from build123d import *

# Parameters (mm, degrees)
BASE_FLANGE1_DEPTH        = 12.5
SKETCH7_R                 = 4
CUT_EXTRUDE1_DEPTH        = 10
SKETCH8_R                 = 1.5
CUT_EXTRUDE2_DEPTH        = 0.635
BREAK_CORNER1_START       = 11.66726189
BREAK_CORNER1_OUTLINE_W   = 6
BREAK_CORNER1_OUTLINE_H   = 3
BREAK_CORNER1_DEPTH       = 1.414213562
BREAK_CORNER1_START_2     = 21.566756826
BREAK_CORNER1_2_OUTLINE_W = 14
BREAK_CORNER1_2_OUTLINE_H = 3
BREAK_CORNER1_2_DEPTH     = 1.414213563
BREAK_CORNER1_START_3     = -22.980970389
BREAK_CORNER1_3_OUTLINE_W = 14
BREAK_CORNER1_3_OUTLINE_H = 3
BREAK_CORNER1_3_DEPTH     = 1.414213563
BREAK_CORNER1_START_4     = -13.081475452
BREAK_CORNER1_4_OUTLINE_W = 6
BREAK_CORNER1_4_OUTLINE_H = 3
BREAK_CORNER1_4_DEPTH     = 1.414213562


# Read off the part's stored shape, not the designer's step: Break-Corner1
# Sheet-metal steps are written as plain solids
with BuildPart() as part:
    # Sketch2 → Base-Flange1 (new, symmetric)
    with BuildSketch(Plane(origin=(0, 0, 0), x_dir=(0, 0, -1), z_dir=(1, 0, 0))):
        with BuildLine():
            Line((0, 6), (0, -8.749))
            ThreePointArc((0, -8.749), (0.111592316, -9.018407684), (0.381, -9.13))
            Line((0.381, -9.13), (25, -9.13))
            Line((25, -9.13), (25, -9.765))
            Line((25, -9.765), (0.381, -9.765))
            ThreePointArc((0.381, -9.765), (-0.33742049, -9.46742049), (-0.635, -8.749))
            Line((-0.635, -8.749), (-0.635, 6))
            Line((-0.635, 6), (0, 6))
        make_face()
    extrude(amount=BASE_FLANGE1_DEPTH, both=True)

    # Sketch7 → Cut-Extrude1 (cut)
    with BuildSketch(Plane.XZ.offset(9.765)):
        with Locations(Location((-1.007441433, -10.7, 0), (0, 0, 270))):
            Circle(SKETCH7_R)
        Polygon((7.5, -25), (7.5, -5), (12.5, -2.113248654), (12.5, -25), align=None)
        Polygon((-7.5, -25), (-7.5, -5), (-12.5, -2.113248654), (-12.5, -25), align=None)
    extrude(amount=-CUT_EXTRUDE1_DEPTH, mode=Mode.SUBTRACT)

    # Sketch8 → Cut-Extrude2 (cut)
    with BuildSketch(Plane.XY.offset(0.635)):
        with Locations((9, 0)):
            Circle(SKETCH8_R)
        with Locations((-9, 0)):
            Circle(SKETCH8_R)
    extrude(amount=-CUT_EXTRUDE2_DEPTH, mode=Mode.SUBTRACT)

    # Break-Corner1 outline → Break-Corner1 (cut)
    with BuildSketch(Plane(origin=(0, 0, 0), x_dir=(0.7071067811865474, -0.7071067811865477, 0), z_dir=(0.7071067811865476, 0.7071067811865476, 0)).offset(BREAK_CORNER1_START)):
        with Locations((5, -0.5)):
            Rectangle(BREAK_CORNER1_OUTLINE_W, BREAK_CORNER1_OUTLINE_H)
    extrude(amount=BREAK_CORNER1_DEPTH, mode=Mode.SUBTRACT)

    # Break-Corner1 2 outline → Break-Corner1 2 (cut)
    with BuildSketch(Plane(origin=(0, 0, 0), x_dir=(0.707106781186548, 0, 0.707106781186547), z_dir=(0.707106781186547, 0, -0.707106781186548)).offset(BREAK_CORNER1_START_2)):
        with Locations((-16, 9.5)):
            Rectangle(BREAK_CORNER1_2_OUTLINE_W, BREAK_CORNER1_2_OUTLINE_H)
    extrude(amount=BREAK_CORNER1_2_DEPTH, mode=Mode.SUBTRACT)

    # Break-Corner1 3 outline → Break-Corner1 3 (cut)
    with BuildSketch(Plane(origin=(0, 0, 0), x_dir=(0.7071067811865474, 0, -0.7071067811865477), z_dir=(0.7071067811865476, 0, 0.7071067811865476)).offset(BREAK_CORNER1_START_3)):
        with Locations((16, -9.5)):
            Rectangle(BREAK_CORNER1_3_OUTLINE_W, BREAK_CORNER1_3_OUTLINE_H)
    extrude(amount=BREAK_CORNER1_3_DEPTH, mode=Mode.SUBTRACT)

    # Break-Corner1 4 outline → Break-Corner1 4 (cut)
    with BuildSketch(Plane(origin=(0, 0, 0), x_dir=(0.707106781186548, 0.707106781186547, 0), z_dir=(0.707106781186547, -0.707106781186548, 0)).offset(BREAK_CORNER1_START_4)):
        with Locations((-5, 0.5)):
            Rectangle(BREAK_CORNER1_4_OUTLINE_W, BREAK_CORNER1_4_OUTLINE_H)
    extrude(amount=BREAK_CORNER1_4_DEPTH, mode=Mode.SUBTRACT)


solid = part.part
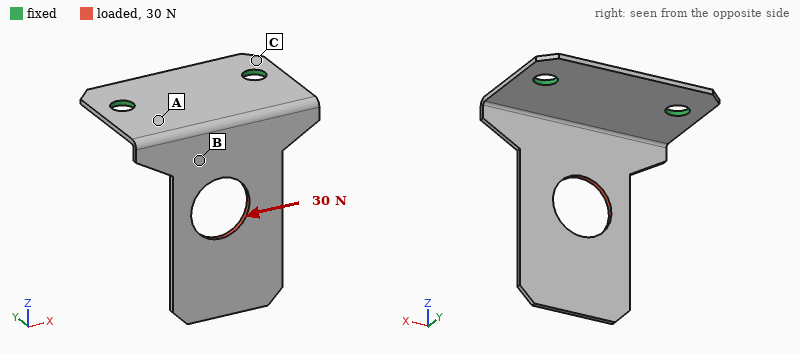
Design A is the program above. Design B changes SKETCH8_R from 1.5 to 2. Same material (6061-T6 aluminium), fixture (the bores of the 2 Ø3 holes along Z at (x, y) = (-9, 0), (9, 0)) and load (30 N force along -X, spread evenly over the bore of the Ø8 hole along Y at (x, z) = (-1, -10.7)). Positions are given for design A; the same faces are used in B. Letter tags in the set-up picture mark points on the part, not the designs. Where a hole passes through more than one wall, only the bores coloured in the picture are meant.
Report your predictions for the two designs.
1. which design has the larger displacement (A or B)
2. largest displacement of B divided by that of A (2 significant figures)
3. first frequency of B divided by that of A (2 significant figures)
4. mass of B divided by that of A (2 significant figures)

A
0.86
1.0
0.98
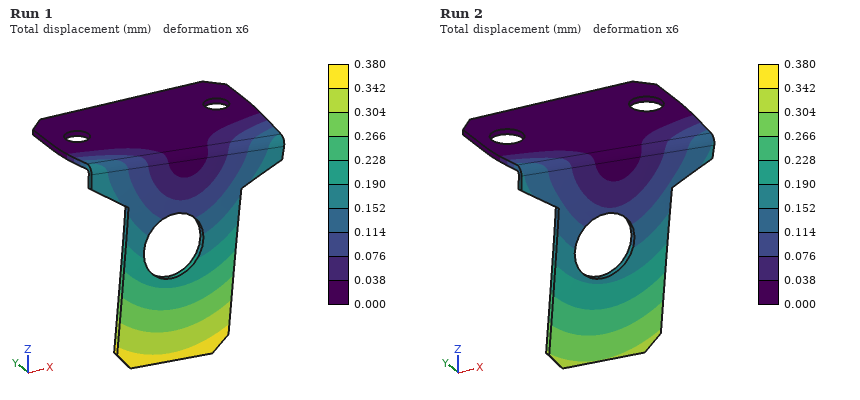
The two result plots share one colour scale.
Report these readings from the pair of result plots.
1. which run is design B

Run 2
